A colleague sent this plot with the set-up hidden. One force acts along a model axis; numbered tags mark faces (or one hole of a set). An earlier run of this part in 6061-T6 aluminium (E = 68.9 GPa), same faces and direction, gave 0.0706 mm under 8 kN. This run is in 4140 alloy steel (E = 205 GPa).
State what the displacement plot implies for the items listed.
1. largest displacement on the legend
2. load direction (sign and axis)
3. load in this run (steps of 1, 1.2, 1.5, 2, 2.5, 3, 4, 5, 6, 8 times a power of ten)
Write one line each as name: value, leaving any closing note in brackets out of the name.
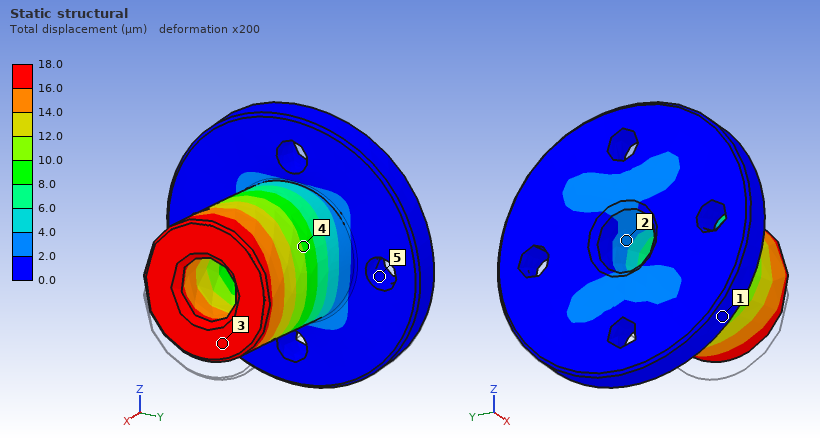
largest displacement on the legend: 18.0 µm
load direction: +Z
load in this run: 6 kN
